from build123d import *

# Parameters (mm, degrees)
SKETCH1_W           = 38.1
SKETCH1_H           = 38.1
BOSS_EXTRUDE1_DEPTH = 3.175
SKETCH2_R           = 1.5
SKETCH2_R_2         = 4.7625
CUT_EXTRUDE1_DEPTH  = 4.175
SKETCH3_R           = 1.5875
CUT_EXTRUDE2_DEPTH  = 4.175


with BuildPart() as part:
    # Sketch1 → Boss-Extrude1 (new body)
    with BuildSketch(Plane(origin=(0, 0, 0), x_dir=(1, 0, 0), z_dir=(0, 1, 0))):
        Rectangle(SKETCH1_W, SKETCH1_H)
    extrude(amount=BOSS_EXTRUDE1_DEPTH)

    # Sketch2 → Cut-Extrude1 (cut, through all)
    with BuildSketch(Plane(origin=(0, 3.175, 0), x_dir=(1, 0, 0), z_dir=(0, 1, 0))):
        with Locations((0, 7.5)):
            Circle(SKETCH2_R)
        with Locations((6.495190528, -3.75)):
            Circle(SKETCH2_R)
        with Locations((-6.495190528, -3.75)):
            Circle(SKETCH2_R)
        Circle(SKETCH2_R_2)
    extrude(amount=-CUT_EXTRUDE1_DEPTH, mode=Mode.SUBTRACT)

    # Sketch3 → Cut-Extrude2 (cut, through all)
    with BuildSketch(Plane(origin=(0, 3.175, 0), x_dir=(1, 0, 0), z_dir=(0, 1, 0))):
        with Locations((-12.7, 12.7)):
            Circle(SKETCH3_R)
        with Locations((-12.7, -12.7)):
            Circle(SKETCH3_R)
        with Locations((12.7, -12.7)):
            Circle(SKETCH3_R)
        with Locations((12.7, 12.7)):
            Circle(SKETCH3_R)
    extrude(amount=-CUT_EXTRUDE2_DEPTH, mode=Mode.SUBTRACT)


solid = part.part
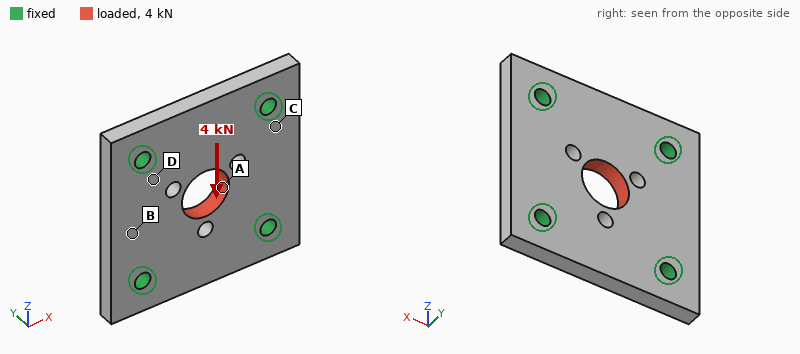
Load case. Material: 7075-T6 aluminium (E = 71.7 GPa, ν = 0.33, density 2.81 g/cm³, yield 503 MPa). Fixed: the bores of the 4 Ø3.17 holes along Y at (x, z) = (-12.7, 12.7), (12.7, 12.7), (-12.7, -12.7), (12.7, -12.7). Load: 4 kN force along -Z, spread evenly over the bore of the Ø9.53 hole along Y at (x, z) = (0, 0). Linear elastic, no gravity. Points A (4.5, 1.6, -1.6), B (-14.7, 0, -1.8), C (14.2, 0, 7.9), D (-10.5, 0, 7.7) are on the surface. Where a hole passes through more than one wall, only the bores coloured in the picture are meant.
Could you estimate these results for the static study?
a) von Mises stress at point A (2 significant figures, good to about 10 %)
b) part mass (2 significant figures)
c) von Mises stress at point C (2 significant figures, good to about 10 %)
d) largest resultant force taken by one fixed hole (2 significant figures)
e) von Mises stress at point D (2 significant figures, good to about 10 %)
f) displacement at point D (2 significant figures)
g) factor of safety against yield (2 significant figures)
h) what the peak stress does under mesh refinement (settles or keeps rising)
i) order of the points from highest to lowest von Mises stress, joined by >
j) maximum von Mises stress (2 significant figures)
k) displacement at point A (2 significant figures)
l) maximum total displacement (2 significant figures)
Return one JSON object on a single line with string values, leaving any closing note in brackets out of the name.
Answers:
{"von Mises stress at point A": "70 MPa", "part mass": "12 g", "von Mises stress at point C": "18 MPa", "largest resultant force taken by one fixed hole": "1.1 kN", "von Mises stress at point D": "33 MPa", "displacement at point D": "2.2 µm", "factor of safety against yield": "3.9", "what the peak stress does under mesh refinement": "settles", "order of the points from highest to lowest von Mises stress, joined by >": "A > D > C > B", "maximum von Mises stress": "130 MPa", "displacement at point A": "9.5 µm", "maximum total displacement": "13 µm"}
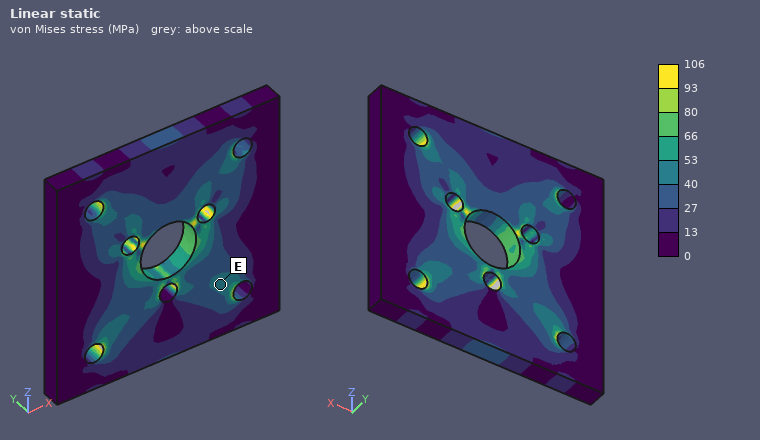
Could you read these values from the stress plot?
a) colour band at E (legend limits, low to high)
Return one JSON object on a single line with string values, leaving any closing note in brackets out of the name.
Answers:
{"colour band at E": "40 to 53 MPa"}
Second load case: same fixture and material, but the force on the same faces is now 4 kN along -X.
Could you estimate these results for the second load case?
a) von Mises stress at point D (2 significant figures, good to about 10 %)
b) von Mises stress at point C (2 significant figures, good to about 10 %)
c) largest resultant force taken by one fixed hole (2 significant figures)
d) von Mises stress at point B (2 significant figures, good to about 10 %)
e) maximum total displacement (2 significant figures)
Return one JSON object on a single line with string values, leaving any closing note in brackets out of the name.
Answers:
{"von Mises stress at point D": "32 MPa", "von Mises stress at point C": "24 MPa", "largest resultant force taken by one fixed hole": "1.1 kN", "von Mises stress at point B": "15 MPa", "maximum total displacement": "12 µm"}
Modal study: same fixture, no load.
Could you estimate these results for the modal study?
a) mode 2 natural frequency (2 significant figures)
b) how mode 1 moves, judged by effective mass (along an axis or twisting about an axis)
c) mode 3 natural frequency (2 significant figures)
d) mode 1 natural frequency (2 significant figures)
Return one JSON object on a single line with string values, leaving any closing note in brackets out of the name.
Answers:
{"mode 2 natural frequency": "24 kHz", "how mode 1 moves, judged by effective mass": "along Y", "mode 3 natural frequency": "25 kHz", "mode 1 natural frequency": "19 kHz"}
